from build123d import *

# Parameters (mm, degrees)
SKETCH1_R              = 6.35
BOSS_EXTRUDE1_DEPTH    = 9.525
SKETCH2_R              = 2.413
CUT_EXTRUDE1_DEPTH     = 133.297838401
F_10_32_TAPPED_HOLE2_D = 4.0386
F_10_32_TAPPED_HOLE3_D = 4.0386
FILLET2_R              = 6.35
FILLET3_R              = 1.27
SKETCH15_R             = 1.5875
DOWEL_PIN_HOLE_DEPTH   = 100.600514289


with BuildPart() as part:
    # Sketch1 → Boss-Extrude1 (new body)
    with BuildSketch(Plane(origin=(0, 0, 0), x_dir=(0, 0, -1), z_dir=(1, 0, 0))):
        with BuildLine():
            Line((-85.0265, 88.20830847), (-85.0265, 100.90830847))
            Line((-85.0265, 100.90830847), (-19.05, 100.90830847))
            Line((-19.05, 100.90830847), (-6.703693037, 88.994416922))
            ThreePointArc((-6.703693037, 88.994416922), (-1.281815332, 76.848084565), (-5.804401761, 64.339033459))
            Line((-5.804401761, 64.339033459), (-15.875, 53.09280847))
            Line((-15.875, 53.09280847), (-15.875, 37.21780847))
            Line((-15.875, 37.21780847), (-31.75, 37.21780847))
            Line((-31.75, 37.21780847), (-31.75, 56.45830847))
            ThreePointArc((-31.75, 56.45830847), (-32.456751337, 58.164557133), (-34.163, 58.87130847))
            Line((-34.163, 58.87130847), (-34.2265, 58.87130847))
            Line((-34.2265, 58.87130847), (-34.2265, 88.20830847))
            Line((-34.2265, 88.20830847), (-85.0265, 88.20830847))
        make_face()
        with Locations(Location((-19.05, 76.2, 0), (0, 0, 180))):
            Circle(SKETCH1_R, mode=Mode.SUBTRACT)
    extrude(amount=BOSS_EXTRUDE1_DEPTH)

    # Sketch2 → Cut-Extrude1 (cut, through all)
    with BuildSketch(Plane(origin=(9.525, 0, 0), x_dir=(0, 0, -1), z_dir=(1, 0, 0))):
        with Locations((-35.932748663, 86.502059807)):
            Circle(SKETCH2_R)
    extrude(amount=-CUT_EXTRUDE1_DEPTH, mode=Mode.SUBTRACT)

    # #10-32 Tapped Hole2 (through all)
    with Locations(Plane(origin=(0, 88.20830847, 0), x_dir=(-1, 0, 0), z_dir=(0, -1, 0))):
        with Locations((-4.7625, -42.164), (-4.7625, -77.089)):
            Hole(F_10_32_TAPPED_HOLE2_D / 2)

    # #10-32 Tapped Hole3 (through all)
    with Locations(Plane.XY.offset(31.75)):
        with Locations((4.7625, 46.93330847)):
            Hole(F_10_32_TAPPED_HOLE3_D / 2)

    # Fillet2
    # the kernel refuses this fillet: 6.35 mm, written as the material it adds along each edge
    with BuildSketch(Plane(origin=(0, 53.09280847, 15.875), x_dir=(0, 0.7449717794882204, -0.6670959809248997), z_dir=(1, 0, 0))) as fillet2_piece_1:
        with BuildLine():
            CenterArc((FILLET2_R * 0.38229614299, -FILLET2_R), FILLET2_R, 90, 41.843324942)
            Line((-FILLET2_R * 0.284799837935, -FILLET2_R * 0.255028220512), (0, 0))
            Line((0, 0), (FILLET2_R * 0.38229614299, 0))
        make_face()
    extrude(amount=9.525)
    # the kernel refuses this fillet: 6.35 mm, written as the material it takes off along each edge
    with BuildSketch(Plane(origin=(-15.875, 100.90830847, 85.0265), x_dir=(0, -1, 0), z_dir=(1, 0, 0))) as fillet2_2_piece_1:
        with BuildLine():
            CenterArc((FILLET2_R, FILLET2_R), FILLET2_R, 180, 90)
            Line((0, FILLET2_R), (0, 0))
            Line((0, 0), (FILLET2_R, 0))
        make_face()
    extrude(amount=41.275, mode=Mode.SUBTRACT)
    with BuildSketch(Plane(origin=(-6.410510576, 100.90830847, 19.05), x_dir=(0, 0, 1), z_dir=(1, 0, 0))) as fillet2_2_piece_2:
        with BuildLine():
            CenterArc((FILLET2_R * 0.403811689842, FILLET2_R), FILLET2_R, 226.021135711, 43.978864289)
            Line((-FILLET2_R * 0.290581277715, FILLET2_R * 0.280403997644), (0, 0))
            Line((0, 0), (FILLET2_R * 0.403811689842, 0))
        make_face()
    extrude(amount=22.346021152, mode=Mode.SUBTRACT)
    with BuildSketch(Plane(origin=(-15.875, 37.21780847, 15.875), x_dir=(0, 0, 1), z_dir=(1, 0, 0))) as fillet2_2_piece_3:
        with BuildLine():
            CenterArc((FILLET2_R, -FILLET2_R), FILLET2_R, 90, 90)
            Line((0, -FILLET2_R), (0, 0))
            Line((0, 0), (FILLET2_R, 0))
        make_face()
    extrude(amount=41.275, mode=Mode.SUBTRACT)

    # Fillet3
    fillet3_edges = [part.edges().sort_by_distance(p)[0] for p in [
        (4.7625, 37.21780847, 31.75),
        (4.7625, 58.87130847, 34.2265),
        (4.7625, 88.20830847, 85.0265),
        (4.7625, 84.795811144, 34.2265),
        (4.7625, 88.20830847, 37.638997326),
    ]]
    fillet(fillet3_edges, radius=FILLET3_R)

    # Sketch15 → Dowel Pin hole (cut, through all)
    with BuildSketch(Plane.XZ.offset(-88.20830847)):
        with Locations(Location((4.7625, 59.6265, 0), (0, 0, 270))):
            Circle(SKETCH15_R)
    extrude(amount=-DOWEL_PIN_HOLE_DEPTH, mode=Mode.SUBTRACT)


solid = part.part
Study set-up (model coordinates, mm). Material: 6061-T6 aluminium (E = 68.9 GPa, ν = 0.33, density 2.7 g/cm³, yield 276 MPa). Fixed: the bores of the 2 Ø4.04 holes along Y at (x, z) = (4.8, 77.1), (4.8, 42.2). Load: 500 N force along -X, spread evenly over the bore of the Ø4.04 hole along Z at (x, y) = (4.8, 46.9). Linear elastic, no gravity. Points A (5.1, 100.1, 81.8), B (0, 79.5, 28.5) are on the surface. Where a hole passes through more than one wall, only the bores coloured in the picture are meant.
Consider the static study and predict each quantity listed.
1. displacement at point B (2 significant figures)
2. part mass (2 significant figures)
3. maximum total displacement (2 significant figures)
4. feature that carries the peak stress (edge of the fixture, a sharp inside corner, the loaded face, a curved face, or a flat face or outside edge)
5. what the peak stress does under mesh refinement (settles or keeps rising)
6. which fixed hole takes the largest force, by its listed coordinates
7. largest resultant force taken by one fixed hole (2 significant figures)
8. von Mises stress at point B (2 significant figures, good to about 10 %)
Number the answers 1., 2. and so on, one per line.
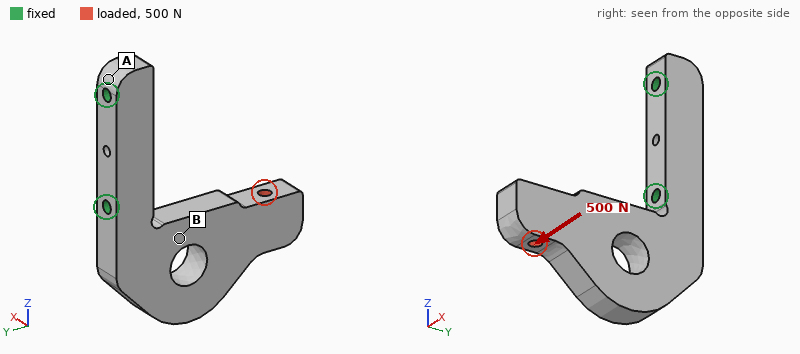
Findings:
1. 0.12 mm
2. 50 g
3. 0.57 mm
4. edge of the fixture
5. keeps rising
6. (4.8, 42.2)
7. 560 N
8. 72 MPa
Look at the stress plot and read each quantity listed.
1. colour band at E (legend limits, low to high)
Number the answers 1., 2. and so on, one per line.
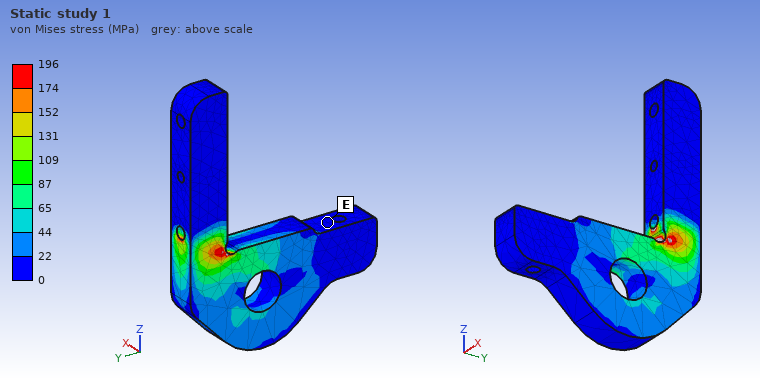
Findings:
1. 0 to 22 MPa
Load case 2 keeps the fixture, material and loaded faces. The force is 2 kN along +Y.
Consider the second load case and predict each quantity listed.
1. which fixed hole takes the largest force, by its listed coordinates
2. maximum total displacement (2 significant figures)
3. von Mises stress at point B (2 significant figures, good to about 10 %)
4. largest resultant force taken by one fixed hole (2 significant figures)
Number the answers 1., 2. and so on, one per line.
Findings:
1. (4.8, 42.2)
2. 0.19 mm
3. 16 MPa
4. 2.1 kN
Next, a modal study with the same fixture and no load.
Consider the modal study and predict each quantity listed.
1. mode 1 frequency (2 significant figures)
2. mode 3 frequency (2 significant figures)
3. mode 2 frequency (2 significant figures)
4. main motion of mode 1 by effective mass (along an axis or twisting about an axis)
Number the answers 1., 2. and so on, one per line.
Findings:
1. 1500 Hz
2. 3700 Hz
3. 2100 Hz
4. along X
